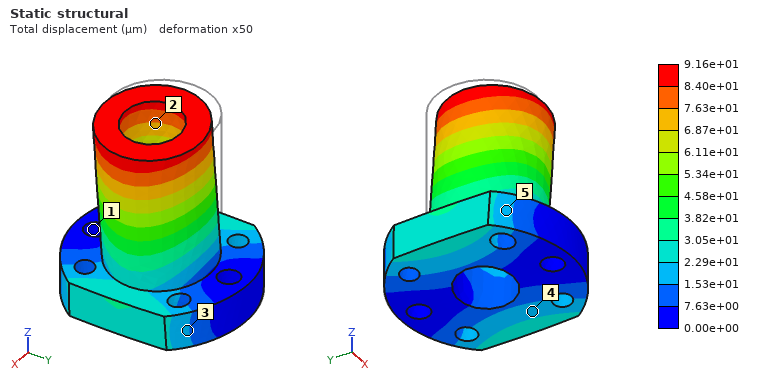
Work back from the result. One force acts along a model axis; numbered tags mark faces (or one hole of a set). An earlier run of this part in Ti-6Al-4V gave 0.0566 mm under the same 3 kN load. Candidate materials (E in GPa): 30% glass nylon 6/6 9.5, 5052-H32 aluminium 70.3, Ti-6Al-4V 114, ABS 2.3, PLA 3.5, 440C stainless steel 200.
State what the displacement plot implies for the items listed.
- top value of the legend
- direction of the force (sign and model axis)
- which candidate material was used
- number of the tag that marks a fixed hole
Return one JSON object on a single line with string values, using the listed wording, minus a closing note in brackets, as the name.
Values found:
{"top value of the legend": "9.16e+01 µm", "direction of the force": "+X", "which candidate material was used": "5052-H32 aluminium", "number of the tag that marks a fixed hole": "1"}
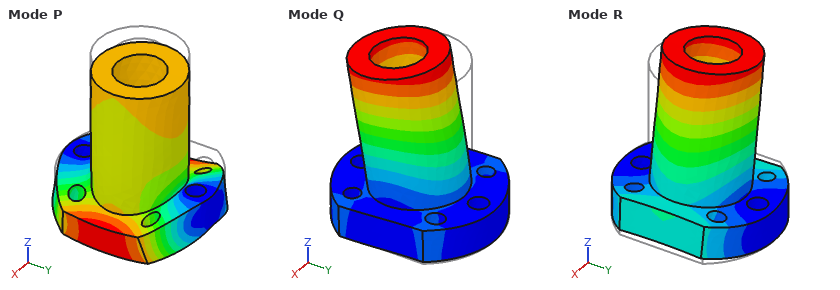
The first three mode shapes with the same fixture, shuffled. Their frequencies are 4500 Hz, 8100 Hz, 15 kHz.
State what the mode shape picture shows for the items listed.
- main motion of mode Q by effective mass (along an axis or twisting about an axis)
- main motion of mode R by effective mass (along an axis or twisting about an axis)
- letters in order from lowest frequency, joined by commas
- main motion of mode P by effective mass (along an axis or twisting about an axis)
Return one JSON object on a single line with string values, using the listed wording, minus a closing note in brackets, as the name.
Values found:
{"main motion of mode Q by effective mass": "along Y", "main motion of mode R by effective mass": "along X", "letters in order from lowest frequency, joined by commas": "R, Q, P", "main motion of mode P by effective mass": "along Z"}
